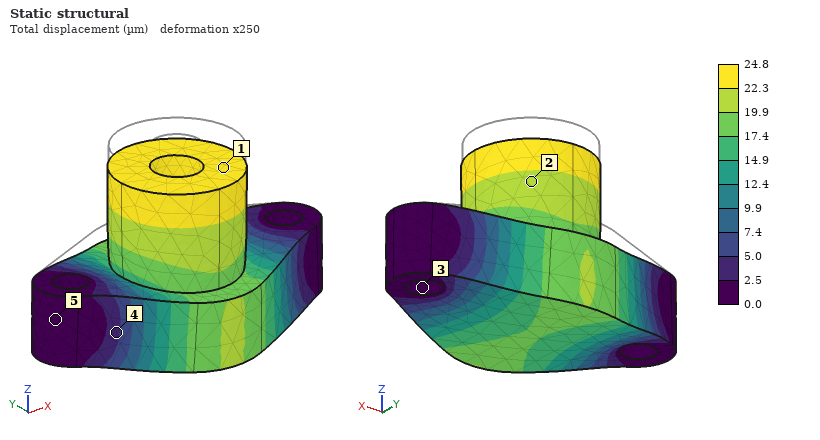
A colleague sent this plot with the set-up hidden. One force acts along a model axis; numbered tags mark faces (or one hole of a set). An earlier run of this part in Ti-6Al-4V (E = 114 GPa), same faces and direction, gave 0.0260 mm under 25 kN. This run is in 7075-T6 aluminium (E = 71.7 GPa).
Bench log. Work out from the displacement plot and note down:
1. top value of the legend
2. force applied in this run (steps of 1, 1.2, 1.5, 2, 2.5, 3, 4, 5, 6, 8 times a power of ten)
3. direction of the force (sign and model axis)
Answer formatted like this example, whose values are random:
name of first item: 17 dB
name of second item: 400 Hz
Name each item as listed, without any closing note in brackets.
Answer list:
top value of the legend: 24.8 µm
force applied in this run: 15 kN
direction of the force: -Z
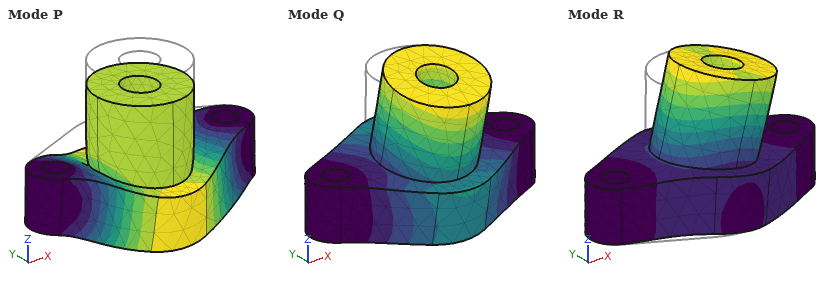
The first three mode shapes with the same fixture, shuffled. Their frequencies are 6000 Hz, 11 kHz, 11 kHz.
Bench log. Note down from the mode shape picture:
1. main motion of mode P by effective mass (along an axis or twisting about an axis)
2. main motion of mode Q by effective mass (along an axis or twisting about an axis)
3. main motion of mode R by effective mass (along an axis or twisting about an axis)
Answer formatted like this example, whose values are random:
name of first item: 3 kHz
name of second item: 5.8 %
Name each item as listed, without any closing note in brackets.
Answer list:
main motion of mode P by effective mass: along Z
main motion of mode Q by effective mass: along Y
main motion of mode R by effective mass: along X
